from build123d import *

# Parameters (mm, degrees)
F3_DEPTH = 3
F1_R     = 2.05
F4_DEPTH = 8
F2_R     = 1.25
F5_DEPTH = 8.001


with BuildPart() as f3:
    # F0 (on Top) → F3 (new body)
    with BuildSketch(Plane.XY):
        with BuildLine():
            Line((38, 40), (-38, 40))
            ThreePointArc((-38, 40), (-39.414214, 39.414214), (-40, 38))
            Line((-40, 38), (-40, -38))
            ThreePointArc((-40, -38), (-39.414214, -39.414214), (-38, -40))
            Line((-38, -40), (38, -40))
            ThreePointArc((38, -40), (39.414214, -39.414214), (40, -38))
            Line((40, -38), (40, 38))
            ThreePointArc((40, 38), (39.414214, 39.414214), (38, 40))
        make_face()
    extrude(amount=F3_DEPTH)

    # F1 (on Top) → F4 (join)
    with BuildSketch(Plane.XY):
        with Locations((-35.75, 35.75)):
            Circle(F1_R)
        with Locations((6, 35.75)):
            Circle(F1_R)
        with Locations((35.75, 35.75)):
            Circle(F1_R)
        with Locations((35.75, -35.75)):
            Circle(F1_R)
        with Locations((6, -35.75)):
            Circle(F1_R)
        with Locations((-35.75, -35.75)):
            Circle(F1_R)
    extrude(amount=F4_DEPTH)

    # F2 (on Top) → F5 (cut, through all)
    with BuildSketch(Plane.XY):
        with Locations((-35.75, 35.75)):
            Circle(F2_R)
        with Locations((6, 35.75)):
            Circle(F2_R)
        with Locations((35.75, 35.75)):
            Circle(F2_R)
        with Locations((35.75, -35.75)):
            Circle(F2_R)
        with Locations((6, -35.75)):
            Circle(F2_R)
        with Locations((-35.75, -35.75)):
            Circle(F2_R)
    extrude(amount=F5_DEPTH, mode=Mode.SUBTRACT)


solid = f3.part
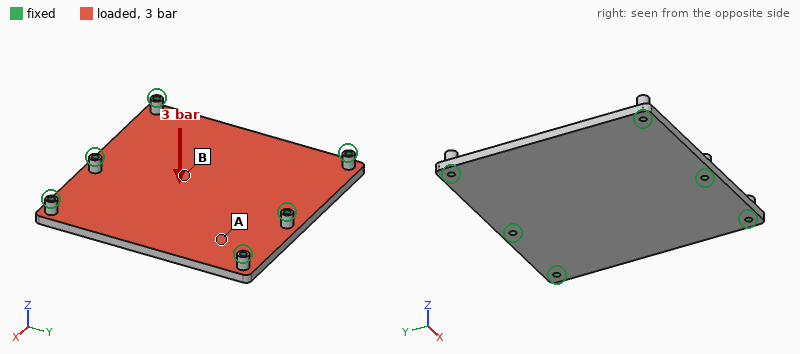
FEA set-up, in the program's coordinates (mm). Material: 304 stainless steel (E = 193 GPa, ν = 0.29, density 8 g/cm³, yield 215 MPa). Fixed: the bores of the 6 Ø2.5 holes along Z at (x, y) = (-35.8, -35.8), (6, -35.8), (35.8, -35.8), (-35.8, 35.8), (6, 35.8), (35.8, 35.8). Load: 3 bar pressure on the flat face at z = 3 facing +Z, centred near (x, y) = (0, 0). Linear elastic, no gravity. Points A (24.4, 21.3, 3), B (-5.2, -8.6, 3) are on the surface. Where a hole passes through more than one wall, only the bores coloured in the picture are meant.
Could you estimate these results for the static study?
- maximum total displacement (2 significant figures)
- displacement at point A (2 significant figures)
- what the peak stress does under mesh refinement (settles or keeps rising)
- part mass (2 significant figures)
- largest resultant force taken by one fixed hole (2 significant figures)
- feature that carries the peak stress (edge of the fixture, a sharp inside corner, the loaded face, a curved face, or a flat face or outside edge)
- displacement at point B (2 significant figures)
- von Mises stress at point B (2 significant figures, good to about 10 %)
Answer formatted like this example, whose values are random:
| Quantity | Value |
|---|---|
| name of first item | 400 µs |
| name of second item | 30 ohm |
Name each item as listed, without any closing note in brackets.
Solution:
| Quantity | Value |
|---|---|
| maximum total displacement | 69 µm |
| displacement at point A | 30 µm |
| what the peak stress does under mesh refinement | keeps rising |
| part mass | 150 g |
| largest resultant force taken by one fixed hole | 440 N |
| feature that carries the peak stress | edge of the fixture |
| displacement at point B | 62 µm |
| von Mises stress at point B | 39 MPa |
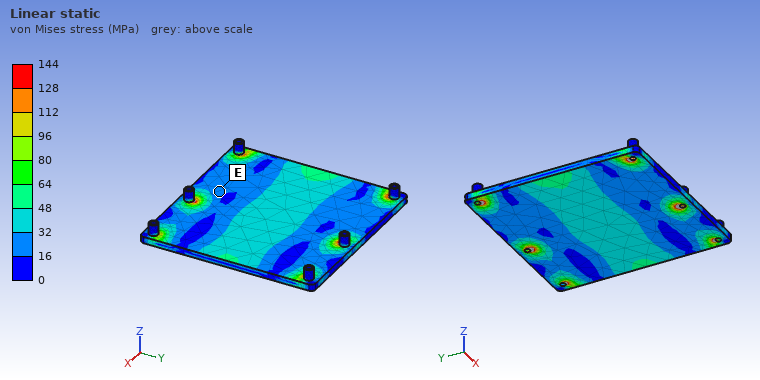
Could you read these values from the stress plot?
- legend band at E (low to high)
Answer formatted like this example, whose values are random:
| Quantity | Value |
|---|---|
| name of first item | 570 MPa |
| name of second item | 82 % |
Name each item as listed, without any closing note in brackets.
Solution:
| Quantity | Value |
|---|---|
| legend band at E | 16 to 32 MPa |
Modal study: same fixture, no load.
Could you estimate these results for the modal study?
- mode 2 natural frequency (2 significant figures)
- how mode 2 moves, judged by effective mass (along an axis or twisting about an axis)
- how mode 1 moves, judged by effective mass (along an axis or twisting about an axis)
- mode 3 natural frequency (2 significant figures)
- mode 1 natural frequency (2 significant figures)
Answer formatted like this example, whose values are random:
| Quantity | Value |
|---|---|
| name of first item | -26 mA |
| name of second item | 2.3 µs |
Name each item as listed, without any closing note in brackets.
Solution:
| Quantity | Value |
|---|---|
| mode 2 natural frequency | 3200 Hz |
| how mode 2 moves, judged by effective mass | twisting about Y |
| how mode 1 moves, judged by effective mass | along Z |
| mode 3 natural frequency | 5100 Hz |
| mode 1 natural frequency | 2500 Hz |
